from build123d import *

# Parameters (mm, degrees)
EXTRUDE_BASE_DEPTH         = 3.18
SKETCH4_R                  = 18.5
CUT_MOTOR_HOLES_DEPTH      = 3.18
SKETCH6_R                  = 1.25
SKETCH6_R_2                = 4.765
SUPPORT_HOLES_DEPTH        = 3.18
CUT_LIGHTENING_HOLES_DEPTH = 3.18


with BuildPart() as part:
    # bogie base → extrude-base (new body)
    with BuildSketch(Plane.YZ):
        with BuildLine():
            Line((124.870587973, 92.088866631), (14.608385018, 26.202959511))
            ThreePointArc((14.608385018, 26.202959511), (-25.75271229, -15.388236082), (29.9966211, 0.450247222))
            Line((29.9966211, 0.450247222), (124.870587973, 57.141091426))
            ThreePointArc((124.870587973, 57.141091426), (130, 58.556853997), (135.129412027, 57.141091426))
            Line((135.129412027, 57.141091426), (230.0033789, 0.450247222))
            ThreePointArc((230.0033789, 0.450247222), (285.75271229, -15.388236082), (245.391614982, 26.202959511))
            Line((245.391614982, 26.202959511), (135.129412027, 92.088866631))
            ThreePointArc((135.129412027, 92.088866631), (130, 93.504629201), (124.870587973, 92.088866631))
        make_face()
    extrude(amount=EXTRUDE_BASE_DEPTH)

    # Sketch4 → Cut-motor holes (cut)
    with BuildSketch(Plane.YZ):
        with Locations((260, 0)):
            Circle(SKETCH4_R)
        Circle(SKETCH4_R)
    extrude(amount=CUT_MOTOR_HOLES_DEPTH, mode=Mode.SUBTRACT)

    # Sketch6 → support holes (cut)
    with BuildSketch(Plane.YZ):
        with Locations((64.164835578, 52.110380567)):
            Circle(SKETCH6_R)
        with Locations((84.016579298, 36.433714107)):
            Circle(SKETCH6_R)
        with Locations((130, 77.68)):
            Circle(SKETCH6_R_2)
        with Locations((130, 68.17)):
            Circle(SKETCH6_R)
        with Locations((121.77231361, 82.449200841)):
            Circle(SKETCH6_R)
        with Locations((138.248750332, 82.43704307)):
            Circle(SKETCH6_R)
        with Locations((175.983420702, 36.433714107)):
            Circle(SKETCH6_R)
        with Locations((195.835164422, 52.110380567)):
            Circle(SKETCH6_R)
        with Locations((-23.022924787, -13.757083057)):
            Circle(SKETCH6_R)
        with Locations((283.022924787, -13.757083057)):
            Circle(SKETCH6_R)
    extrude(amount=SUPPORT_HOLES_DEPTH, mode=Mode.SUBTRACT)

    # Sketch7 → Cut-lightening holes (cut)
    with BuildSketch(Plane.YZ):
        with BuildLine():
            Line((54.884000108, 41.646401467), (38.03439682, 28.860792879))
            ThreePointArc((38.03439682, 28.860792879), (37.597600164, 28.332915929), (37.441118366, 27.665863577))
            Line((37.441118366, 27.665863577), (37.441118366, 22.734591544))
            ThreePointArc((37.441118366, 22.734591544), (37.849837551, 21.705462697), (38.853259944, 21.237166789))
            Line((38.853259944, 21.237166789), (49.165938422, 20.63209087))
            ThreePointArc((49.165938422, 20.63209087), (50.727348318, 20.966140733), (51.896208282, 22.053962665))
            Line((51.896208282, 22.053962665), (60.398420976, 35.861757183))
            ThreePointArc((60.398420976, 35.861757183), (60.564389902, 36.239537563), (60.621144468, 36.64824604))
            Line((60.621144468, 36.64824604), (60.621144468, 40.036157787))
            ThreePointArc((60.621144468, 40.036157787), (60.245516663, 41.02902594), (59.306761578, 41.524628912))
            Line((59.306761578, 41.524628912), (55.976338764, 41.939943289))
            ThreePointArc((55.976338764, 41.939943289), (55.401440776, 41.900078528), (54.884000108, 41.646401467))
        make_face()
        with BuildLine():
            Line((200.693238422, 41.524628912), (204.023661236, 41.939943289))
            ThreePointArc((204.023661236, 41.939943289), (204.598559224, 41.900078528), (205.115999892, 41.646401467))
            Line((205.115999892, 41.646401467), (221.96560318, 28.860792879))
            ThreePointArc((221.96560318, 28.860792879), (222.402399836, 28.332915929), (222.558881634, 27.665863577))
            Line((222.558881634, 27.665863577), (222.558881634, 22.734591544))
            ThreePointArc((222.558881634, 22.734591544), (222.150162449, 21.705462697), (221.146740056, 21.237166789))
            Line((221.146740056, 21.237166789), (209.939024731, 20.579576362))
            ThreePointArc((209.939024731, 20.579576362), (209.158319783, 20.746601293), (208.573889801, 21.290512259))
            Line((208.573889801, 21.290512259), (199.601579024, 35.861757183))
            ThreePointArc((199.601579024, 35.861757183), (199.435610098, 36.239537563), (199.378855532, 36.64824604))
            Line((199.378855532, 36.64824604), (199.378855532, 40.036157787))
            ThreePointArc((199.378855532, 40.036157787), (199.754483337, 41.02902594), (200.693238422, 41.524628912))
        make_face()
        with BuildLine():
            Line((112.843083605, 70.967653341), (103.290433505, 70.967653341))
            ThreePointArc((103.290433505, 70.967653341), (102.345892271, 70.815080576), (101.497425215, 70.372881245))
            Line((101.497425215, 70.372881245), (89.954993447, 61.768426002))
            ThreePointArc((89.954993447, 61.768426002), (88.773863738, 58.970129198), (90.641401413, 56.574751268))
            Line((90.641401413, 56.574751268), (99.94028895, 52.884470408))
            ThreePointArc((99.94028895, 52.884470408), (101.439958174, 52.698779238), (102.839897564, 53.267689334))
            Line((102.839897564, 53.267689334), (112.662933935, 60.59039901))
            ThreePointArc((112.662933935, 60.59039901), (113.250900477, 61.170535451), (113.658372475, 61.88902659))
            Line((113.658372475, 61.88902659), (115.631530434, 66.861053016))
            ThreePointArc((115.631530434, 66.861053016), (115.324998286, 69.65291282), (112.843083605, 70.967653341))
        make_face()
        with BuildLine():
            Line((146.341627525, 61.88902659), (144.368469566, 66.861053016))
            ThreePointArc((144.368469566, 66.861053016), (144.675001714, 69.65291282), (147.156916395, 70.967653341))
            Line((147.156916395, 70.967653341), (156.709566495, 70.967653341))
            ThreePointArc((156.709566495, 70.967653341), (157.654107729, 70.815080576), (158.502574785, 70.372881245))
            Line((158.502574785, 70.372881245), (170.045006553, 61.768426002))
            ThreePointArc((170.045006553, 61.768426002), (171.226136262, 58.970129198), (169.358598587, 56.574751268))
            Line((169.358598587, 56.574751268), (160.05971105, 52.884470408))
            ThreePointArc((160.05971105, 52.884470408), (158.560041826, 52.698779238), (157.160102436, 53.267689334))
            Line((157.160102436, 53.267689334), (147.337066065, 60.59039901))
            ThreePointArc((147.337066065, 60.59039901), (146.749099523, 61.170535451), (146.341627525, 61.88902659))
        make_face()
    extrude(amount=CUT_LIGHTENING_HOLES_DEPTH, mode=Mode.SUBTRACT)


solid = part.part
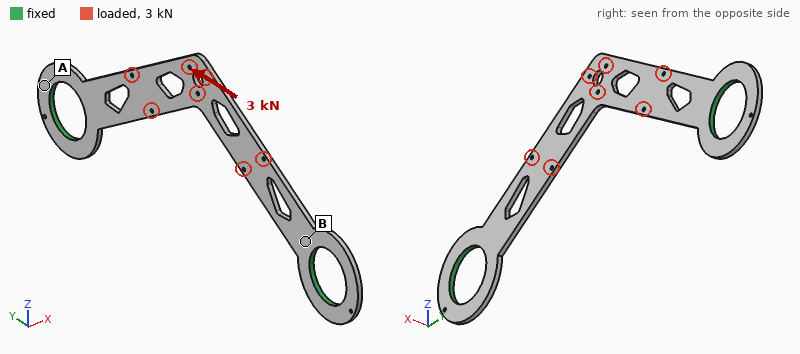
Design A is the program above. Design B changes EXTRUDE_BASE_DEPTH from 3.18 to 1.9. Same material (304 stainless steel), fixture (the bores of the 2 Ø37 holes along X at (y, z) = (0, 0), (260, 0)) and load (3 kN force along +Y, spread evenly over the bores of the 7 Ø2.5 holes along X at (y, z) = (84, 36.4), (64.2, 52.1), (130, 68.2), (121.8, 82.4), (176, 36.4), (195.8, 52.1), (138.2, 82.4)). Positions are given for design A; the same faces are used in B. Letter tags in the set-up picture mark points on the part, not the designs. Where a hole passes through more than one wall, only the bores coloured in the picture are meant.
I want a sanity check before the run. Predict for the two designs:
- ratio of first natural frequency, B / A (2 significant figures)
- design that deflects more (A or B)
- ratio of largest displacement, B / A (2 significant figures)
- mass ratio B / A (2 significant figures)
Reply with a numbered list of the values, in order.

1. 0.60
2. B
3. 1.7
4. 0.60
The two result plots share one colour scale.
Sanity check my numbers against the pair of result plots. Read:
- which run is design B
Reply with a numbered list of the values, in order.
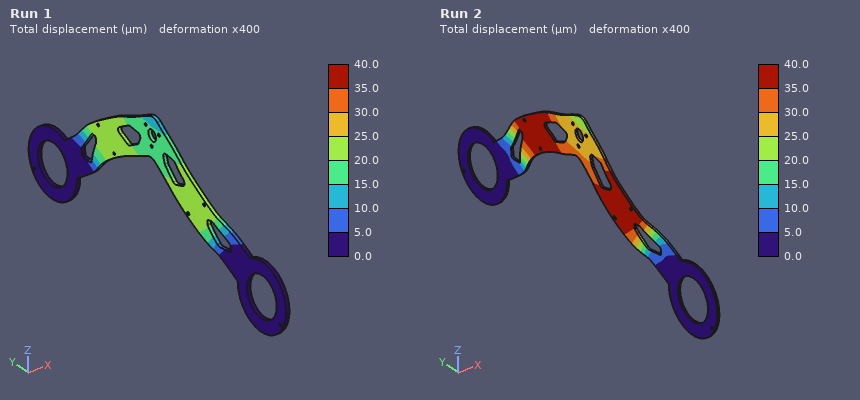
1. Run 2
